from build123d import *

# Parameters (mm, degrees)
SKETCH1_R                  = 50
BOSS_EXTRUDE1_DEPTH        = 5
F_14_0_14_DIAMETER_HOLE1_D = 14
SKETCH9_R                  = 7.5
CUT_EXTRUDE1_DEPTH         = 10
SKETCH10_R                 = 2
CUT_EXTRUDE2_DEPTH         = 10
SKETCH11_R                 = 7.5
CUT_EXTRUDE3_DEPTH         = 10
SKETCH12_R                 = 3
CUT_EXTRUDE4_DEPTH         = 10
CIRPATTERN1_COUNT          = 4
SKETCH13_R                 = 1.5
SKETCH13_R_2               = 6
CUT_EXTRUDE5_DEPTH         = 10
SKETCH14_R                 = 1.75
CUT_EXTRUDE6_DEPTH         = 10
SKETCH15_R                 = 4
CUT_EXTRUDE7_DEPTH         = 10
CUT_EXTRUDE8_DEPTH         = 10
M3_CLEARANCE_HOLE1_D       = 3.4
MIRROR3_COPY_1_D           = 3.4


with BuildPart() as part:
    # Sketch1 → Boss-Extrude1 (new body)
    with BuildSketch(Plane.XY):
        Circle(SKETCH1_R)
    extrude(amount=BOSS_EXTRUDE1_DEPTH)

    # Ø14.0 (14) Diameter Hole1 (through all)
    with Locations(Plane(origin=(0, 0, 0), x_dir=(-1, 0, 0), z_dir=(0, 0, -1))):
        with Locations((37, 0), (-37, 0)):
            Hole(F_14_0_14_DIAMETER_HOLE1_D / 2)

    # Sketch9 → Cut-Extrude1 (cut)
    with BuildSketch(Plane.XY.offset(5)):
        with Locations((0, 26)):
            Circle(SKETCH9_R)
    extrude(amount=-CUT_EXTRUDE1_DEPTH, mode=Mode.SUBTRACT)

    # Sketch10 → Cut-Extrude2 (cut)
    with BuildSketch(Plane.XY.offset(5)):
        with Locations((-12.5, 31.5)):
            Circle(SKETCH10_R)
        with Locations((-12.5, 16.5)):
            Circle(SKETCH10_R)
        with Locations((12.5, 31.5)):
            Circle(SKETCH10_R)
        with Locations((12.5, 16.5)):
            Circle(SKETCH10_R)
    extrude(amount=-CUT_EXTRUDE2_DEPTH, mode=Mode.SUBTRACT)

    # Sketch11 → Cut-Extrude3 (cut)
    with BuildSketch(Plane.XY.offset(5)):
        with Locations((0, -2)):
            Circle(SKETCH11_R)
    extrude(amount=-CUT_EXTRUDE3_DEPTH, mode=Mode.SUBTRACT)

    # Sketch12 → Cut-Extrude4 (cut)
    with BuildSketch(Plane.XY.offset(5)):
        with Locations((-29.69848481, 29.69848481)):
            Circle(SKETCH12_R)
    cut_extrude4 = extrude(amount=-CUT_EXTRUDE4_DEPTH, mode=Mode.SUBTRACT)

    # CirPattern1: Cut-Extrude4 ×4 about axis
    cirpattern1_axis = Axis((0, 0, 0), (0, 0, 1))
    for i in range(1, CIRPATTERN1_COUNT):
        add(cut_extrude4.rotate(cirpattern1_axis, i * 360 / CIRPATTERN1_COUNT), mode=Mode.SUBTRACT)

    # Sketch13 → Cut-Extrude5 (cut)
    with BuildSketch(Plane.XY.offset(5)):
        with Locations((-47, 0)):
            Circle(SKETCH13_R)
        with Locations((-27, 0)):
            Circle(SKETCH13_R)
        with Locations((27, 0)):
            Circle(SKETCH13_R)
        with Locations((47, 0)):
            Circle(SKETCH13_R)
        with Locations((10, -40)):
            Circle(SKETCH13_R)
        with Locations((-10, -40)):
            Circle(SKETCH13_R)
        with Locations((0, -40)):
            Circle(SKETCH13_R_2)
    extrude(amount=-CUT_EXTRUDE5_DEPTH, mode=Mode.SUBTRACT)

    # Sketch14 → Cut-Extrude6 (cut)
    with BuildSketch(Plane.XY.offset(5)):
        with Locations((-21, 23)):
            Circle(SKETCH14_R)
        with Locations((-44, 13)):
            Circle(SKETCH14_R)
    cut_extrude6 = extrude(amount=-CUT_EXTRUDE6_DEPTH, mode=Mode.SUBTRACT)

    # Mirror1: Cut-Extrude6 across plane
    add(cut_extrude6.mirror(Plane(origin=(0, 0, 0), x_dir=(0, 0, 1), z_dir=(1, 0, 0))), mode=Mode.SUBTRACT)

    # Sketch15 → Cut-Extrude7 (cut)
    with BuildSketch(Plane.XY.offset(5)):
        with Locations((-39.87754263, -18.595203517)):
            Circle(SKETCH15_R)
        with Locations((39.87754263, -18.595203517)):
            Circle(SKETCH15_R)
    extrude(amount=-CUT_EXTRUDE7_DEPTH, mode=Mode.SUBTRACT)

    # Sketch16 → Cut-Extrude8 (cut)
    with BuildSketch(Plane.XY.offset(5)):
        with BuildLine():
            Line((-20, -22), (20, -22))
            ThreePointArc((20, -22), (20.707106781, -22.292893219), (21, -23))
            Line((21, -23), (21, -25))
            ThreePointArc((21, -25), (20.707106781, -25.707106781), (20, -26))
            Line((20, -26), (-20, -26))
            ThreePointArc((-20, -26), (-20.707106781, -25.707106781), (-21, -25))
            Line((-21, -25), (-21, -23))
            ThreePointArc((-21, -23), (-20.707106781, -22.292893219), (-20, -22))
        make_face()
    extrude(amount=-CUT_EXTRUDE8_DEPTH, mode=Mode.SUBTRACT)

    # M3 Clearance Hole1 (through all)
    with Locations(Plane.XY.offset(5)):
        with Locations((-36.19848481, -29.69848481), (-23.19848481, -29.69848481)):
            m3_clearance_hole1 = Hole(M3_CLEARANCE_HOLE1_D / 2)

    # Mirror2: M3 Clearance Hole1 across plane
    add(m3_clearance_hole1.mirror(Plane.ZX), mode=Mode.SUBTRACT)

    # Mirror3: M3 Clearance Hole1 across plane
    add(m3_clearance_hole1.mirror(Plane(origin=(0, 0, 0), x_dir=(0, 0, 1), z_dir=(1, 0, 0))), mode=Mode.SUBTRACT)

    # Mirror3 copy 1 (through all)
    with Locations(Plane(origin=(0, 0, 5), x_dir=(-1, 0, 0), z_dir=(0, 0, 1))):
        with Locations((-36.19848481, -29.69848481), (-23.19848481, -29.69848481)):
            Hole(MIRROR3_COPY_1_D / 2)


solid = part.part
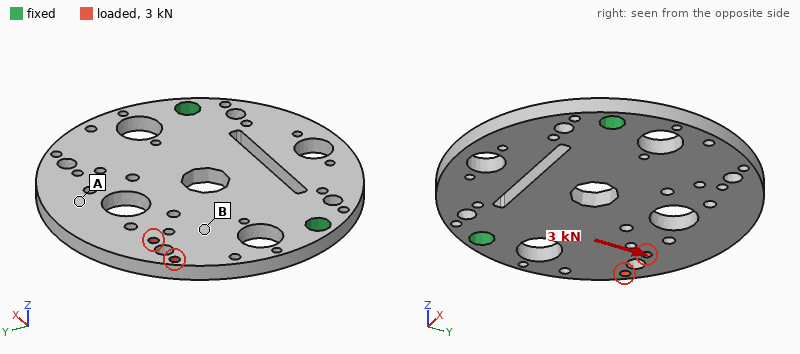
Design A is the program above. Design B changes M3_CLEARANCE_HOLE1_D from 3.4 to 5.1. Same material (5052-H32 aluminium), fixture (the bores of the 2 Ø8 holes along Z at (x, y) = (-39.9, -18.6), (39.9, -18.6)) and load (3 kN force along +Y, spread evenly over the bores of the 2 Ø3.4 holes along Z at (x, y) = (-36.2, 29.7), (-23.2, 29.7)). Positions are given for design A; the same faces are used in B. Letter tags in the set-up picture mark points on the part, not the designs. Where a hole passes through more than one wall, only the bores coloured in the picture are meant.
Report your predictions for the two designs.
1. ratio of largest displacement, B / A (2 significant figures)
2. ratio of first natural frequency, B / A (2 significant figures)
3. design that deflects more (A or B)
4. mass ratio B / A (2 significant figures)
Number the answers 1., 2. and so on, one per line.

1. 1.1
2. 1.0
3. B
4. 0.99
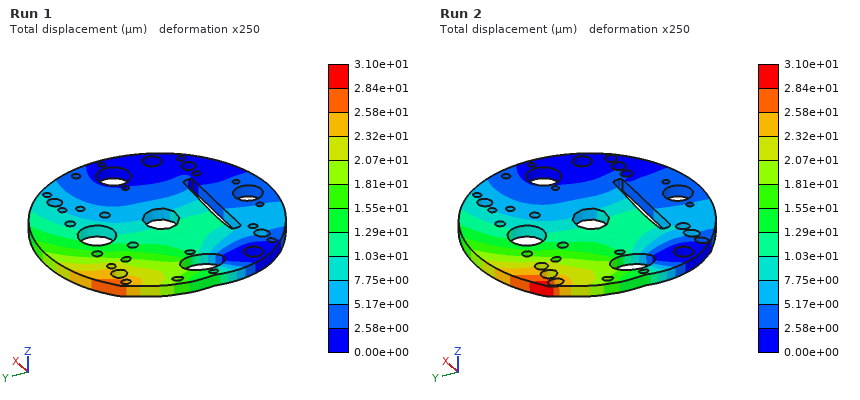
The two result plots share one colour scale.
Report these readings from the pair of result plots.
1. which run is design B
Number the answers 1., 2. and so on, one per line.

1. Run 2
